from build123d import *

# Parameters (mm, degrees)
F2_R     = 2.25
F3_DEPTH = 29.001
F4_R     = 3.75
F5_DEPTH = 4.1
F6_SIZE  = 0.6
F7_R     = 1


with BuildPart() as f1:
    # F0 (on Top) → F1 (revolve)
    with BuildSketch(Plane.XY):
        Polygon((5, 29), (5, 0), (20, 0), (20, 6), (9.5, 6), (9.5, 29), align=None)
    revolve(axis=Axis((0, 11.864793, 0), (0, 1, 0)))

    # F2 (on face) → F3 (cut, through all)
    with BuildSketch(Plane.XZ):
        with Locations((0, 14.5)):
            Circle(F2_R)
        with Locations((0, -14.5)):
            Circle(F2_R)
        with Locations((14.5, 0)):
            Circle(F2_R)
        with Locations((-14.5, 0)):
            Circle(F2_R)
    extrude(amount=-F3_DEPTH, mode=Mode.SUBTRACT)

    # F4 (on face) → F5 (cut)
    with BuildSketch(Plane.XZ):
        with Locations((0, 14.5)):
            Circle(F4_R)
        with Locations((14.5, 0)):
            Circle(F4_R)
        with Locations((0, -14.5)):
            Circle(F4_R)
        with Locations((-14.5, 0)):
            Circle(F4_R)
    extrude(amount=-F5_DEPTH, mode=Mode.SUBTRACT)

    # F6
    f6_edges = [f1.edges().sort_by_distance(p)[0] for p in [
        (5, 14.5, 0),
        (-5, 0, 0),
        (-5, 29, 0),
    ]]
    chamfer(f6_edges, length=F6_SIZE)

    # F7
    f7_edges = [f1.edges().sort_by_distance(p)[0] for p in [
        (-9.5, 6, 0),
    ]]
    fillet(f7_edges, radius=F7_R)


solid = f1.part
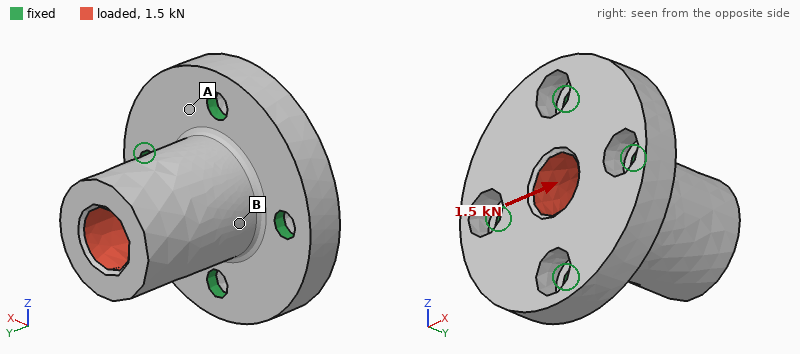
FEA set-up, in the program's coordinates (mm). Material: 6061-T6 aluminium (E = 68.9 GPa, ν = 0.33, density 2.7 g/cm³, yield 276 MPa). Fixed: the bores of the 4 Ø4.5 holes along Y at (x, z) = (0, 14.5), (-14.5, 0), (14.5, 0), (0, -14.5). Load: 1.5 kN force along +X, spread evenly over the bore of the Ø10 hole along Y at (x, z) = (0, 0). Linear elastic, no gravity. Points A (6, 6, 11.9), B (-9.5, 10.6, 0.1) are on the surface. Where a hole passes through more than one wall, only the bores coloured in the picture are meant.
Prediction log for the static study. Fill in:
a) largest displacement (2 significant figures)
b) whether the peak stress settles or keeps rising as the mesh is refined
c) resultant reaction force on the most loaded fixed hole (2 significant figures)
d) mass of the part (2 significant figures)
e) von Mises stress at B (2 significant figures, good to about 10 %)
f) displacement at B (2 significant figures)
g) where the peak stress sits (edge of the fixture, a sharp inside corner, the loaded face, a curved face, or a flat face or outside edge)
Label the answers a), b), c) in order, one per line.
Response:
a) 21 µm
b) keeps rising
c) 620 N
d) 30 g
e) 14 MPa
f) 7.8 µm
g) edge of the fixture
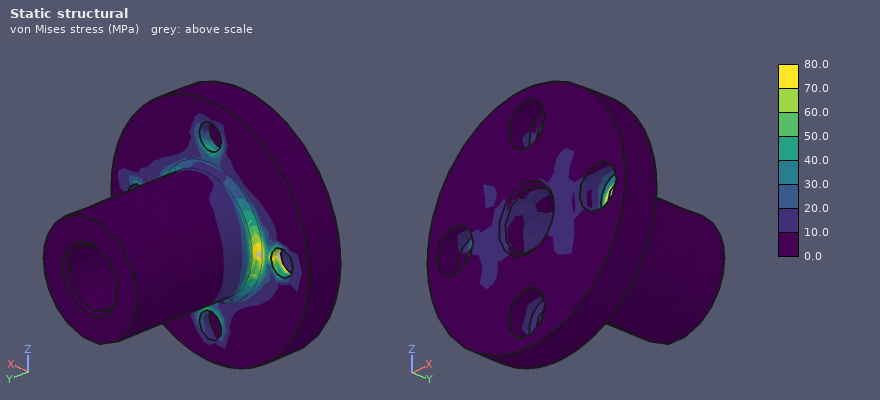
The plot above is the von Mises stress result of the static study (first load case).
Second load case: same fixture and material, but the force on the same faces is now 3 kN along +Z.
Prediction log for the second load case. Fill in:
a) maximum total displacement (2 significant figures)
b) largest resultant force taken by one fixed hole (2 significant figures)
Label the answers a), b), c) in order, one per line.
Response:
a) 42 µm
b) 1.2 kN
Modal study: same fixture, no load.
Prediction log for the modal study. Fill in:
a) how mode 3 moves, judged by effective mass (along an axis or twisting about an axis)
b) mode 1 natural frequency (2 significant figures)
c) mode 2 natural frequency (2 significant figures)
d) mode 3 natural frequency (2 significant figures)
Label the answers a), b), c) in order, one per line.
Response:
a) along Y
b) 12 kHz
c) 12 kHz
d) 22 kHz
